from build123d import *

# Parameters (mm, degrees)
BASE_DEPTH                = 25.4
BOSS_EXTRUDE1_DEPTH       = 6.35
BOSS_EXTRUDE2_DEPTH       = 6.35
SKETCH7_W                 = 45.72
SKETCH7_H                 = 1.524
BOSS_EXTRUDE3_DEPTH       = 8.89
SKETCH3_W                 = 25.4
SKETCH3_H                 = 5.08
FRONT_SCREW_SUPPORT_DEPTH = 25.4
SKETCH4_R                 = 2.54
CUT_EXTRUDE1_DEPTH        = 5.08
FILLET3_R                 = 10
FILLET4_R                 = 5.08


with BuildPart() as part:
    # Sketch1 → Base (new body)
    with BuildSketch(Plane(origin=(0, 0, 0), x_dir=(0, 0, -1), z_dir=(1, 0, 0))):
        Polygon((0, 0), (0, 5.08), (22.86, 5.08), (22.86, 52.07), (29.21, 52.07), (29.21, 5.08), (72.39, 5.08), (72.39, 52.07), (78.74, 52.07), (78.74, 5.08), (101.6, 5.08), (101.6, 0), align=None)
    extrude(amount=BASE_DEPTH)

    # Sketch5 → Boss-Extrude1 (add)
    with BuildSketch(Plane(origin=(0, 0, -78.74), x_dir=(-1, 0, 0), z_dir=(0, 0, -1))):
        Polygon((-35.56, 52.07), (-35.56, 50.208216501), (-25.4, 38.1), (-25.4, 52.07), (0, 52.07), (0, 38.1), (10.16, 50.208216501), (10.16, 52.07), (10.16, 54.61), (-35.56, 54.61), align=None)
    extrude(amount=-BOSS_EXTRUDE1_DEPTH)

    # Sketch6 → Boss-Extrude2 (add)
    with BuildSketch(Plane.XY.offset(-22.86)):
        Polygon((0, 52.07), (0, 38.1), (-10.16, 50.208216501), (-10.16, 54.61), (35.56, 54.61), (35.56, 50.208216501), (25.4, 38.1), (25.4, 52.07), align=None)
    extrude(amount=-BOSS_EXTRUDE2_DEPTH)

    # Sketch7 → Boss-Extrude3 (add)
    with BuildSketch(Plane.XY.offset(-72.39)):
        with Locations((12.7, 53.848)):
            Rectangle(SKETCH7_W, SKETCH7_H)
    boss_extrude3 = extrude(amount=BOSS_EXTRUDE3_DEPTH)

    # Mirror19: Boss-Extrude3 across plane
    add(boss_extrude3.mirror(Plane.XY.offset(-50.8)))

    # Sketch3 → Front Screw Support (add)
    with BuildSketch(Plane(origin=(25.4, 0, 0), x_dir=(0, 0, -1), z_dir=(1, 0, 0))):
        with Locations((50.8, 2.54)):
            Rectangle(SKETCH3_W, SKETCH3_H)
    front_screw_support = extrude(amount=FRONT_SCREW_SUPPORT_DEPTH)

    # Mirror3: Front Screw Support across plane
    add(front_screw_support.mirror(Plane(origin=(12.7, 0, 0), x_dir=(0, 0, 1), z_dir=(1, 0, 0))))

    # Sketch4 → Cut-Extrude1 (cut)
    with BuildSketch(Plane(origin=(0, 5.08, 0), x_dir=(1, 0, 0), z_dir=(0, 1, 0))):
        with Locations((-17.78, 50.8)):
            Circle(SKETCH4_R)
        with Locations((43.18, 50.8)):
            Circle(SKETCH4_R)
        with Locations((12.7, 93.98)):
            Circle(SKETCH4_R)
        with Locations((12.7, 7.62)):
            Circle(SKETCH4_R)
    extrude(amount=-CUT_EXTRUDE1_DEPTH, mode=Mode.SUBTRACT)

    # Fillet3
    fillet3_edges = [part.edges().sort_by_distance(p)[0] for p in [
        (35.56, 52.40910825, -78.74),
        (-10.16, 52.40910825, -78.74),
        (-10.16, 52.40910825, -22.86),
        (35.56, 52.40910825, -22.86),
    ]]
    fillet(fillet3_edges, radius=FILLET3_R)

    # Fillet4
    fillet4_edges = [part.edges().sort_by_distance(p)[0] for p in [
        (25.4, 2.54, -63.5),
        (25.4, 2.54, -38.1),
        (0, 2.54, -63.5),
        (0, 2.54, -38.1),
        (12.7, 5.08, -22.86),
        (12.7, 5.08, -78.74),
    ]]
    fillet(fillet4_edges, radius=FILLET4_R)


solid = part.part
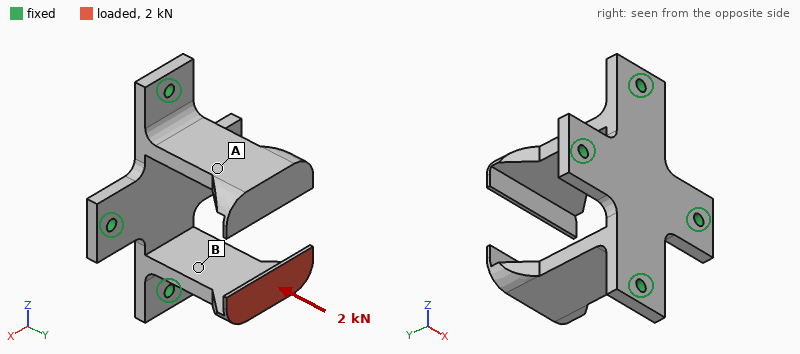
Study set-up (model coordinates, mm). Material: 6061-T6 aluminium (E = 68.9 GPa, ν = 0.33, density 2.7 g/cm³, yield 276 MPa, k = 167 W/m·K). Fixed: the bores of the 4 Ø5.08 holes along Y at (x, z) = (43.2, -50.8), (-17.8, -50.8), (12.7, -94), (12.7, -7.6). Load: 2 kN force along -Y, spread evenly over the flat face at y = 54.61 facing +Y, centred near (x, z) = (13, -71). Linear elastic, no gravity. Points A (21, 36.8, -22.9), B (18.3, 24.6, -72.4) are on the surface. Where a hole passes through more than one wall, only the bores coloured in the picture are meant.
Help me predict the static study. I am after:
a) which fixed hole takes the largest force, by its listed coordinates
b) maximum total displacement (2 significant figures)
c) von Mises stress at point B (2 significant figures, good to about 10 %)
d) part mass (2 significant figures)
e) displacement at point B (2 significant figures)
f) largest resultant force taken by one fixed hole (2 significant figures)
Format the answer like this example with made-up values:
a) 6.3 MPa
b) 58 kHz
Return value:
a) (12.7, -94)
b) 0.65 mm
c) 68 MPa
d) 110 g
e) 0.15 mm
f) 1.0 kN
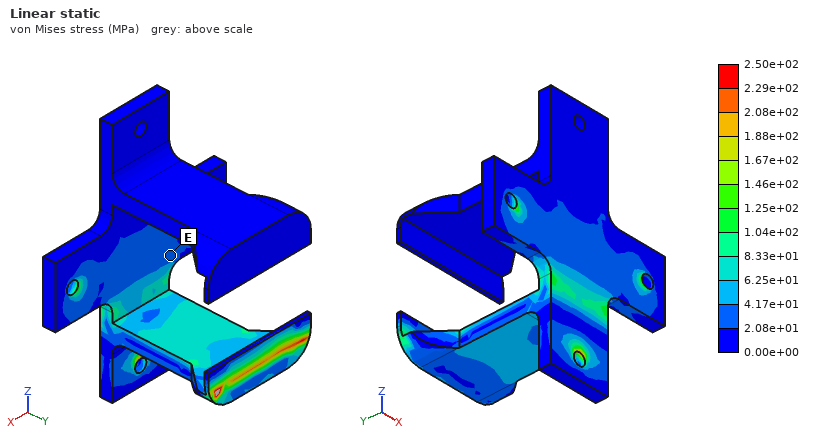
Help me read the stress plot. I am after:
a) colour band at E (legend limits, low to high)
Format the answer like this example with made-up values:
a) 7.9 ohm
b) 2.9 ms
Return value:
a) 2.08e+01 to 4.17e+01 MPa
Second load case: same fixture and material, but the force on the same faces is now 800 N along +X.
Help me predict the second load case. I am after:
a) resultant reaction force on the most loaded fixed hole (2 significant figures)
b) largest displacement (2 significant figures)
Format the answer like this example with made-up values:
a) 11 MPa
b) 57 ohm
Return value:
a) 610 N
b) 0.58 mm
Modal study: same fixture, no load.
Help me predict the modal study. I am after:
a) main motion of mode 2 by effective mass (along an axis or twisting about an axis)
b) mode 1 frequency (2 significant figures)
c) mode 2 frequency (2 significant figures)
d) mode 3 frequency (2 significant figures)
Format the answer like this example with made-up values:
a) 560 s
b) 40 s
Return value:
a) along Z
b) 1300 Hz
c) 1400 Hz
d) 1800 Hz
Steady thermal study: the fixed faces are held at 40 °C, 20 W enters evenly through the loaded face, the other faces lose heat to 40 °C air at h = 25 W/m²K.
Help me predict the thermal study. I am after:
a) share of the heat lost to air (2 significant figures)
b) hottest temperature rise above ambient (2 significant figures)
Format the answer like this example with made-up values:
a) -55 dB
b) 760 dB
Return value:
a) 16 %
b) 45 K
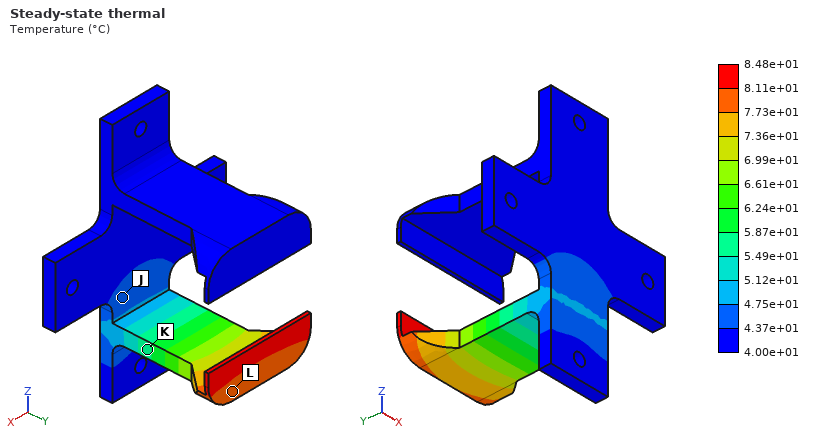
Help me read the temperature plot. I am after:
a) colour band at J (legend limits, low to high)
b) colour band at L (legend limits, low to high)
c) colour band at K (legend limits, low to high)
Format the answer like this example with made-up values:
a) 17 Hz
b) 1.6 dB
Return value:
a) 4.37e+01 to 4.75e+01 °C
b) 7.73e+01 to 8.11e+01 °C
c) 5.49e+01 to 5.87e+01 °C
